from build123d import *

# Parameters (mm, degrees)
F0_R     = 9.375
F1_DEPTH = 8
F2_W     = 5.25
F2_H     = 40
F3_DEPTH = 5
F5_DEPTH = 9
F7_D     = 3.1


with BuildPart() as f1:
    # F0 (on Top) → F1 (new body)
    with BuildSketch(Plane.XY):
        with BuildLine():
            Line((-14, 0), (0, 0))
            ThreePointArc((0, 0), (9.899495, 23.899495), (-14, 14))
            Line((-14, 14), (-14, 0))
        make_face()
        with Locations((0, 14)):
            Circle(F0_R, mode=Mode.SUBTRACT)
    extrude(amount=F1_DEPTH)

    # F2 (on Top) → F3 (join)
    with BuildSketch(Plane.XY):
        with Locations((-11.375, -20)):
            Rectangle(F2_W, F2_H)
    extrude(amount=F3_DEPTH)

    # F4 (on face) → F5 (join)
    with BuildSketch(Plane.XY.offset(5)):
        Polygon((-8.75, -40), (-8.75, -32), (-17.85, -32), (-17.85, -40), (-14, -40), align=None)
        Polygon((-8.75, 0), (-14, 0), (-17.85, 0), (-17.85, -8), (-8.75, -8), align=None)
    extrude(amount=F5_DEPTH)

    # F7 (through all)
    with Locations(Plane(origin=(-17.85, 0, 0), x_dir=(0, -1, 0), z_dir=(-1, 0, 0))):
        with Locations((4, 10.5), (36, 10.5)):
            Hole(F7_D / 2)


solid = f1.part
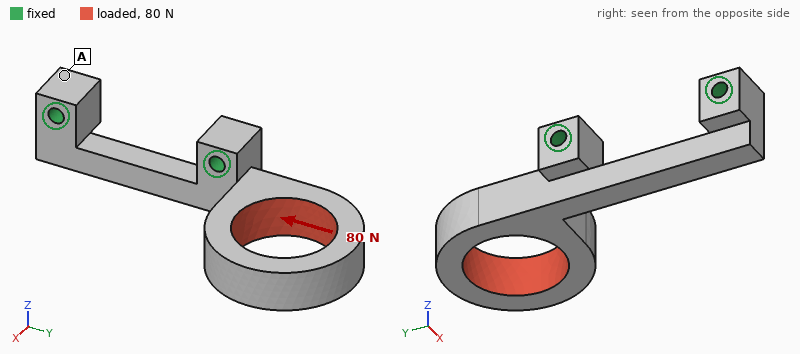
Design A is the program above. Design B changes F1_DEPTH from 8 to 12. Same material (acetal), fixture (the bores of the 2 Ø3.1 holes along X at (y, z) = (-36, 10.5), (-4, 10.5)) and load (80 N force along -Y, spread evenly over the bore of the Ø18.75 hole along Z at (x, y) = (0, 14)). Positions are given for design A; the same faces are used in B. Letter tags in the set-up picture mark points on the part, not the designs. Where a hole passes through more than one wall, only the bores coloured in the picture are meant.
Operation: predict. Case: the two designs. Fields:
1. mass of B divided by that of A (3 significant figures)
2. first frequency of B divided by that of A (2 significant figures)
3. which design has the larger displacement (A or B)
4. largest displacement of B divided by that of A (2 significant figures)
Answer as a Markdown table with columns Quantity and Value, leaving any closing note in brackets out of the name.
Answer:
| Quantity | Value |
|---|---|
| mass of B divided by that of A | 1.29 |
| first frequency of B divided by that of A | 1.1 |
| which design has the larger displacement | A |
| largest displacement of B divided by that of A | 0.60 |
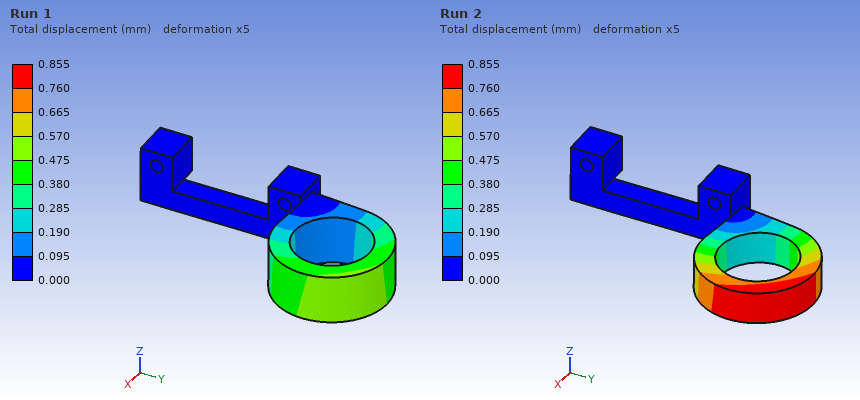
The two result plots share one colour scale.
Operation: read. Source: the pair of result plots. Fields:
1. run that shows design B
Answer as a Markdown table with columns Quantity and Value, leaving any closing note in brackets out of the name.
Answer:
| Quantity | Value |
|---|---|
| run that shows design B | Run 1 |
